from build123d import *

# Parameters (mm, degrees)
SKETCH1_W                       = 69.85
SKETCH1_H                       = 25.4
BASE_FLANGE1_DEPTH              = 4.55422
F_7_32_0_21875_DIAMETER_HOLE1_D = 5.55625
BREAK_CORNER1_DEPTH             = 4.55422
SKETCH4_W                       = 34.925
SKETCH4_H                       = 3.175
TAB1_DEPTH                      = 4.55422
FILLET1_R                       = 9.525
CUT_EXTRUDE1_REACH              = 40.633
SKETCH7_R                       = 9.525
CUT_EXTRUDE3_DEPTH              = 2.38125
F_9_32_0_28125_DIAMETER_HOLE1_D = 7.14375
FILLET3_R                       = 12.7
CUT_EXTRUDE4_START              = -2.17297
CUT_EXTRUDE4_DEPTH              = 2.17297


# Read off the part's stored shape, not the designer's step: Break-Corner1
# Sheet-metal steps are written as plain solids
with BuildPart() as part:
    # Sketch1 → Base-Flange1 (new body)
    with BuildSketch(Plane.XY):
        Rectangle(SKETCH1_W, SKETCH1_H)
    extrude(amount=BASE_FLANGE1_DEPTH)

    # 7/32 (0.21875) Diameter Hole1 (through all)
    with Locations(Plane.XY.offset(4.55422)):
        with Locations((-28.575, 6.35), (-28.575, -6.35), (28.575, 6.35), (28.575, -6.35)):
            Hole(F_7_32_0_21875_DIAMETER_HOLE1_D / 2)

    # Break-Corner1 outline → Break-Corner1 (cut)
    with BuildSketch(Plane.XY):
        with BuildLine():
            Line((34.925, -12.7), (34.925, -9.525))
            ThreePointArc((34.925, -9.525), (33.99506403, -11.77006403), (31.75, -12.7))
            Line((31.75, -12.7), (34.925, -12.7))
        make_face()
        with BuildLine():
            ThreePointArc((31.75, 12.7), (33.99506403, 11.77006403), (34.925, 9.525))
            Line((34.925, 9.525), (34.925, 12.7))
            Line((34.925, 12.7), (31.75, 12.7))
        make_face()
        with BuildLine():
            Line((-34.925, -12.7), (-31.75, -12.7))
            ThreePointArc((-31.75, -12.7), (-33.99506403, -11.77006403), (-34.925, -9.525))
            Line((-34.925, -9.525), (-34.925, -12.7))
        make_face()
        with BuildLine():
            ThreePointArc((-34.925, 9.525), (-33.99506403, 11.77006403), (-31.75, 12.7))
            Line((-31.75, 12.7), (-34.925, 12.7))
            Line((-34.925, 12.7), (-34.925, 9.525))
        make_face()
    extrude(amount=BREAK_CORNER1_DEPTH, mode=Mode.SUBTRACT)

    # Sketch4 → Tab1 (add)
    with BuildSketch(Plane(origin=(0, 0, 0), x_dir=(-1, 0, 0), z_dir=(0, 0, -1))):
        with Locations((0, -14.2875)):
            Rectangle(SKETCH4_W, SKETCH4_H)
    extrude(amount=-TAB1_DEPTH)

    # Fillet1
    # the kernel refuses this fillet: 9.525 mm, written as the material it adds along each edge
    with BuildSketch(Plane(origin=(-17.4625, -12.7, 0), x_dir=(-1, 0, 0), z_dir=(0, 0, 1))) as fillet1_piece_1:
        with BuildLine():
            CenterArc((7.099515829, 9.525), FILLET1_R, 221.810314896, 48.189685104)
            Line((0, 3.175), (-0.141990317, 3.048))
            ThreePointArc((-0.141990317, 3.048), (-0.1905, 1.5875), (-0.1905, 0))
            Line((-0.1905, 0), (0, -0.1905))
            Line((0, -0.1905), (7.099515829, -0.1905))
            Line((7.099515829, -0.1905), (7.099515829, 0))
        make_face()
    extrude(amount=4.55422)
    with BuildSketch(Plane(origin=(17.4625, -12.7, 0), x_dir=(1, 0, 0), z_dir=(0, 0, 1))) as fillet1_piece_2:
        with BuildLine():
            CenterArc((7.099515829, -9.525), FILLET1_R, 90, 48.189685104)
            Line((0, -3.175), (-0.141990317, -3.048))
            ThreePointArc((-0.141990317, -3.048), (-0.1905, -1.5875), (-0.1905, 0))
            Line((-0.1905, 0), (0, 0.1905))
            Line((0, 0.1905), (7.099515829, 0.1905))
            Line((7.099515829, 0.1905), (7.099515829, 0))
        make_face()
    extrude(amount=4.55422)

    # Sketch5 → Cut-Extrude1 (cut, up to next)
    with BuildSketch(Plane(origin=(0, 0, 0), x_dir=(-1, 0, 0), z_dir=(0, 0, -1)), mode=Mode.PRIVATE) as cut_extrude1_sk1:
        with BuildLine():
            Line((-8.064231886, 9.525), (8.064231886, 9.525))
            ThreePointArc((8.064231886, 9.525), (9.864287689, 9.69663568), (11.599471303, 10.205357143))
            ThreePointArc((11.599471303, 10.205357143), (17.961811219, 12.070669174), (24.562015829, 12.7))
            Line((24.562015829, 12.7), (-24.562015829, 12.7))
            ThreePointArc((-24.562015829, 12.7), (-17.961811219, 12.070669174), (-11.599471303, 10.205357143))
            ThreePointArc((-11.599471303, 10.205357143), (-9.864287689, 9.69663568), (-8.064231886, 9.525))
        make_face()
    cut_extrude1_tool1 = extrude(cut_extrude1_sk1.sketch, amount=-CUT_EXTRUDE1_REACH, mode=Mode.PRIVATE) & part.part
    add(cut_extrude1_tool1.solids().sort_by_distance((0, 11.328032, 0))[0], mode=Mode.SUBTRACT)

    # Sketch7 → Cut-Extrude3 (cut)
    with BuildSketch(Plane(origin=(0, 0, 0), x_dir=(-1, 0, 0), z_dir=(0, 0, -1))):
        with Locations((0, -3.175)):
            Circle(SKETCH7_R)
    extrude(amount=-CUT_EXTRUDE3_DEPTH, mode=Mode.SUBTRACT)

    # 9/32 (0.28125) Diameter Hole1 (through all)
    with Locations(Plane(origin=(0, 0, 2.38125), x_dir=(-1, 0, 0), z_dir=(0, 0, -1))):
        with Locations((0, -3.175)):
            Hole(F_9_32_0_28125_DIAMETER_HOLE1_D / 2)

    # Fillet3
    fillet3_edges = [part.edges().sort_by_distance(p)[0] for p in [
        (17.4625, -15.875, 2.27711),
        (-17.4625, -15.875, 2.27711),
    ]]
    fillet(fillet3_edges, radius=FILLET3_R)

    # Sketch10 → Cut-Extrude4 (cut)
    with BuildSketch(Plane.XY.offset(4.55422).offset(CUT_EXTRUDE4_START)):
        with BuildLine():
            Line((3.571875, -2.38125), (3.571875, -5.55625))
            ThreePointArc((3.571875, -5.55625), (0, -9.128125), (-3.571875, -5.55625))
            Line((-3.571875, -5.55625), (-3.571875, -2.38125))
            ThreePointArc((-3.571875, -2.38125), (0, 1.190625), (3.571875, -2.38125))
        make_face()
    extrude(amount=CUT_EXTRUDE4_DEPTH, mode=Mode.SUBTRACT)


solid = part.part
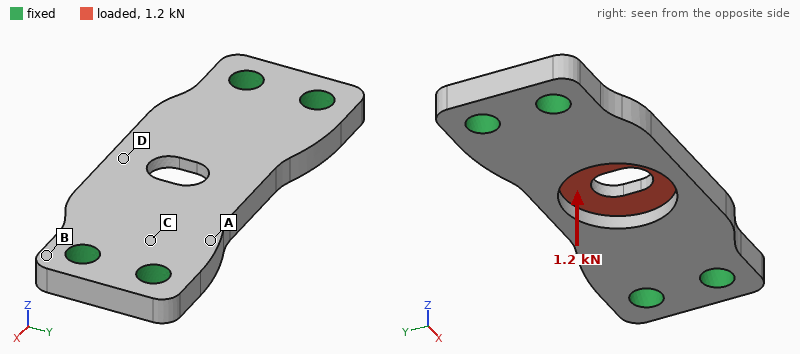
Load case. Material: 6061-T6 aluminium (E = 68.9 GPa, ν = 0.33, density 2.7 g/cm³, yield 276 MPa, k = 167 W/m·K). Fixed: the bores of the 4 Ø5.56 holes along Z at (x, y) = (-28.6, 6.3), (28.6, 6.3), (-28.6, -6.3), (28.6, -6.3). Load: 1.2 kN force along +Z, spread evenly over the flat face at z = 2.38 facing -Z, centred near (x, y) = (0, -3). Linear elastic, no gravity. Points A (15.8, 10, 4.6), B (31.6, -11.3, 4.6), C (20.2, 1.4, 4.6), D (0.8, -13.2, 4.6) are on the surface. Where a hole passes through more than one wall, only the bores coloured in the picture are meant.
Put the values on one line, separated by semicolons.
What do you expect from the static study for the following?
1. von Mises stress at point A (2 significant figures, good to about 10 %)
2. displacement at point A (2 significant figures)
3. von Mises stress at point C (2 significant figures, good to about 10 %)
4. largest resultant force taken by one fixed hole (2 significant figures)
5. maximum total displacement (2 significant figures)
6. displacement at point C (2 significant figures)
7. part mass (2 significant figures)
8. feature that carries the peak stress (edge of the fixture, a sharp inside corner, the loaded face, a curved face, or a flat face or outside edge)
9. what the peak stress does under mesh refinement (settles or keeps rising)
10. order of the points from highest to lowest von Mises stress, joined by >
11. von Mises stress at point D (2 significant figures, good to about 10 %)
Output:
29 MPa; 0.027 mm; 49 MPa; 490 N; 0.11 mm; 0.016 mm; 19 g; edge of the fixture; keeps rising; D > C > A > B; 100 MPa
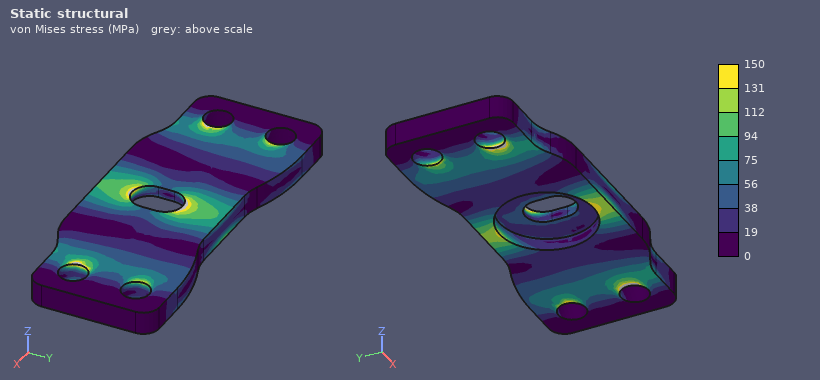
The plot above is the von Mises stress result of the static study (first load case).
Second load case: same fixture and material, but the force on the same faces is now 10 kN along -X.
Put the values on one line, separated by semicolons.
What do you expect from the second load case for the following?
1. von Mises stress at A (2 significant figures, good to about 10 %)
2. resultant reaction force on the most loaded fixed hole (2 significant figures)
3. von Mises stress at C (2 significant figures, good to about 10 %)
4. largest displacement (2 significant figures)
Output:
37 MPa; 2.9 kN; 55 MPa; 29 µm
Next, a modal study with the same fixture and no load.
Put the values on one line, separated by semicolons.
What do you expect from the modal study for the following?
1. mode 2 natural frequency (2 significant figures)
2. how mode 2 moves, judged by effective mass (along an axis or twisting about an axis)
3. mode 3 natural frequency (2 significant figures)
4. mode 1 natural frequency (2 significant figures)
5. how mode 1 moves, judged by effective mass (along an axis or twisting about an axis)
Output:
12 kHz; twisting about X; 18 kHz; 8100 Hz; along Z
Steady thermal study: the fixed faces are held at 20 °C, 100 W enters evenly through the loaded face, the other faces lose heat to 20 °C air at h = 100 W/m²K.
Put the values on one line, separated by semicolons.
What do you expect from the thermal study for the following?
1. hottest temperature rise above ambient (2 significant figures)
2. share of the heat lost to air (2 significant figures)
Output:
68 K; 9.7 %
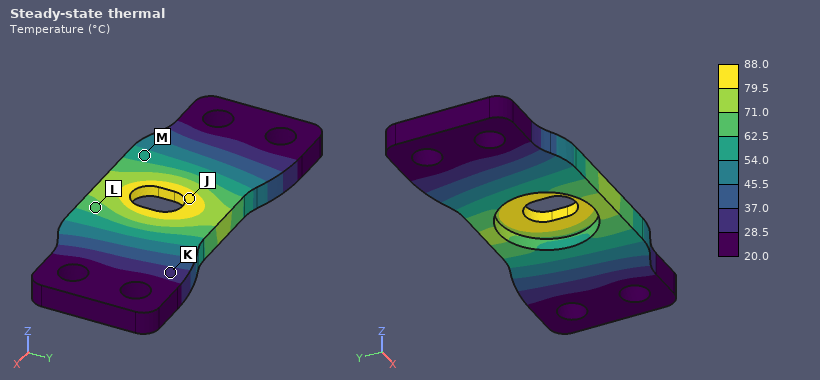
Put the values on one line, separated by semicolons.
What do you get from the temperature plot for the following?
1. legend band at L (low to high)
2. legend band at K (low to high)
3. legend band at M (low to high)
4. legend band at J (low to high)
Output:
62.5 to 71.0 °C; 28.5 to 37.0 °C; 54.0 to 62.5 °C; 79.5 to 88.0 °C
